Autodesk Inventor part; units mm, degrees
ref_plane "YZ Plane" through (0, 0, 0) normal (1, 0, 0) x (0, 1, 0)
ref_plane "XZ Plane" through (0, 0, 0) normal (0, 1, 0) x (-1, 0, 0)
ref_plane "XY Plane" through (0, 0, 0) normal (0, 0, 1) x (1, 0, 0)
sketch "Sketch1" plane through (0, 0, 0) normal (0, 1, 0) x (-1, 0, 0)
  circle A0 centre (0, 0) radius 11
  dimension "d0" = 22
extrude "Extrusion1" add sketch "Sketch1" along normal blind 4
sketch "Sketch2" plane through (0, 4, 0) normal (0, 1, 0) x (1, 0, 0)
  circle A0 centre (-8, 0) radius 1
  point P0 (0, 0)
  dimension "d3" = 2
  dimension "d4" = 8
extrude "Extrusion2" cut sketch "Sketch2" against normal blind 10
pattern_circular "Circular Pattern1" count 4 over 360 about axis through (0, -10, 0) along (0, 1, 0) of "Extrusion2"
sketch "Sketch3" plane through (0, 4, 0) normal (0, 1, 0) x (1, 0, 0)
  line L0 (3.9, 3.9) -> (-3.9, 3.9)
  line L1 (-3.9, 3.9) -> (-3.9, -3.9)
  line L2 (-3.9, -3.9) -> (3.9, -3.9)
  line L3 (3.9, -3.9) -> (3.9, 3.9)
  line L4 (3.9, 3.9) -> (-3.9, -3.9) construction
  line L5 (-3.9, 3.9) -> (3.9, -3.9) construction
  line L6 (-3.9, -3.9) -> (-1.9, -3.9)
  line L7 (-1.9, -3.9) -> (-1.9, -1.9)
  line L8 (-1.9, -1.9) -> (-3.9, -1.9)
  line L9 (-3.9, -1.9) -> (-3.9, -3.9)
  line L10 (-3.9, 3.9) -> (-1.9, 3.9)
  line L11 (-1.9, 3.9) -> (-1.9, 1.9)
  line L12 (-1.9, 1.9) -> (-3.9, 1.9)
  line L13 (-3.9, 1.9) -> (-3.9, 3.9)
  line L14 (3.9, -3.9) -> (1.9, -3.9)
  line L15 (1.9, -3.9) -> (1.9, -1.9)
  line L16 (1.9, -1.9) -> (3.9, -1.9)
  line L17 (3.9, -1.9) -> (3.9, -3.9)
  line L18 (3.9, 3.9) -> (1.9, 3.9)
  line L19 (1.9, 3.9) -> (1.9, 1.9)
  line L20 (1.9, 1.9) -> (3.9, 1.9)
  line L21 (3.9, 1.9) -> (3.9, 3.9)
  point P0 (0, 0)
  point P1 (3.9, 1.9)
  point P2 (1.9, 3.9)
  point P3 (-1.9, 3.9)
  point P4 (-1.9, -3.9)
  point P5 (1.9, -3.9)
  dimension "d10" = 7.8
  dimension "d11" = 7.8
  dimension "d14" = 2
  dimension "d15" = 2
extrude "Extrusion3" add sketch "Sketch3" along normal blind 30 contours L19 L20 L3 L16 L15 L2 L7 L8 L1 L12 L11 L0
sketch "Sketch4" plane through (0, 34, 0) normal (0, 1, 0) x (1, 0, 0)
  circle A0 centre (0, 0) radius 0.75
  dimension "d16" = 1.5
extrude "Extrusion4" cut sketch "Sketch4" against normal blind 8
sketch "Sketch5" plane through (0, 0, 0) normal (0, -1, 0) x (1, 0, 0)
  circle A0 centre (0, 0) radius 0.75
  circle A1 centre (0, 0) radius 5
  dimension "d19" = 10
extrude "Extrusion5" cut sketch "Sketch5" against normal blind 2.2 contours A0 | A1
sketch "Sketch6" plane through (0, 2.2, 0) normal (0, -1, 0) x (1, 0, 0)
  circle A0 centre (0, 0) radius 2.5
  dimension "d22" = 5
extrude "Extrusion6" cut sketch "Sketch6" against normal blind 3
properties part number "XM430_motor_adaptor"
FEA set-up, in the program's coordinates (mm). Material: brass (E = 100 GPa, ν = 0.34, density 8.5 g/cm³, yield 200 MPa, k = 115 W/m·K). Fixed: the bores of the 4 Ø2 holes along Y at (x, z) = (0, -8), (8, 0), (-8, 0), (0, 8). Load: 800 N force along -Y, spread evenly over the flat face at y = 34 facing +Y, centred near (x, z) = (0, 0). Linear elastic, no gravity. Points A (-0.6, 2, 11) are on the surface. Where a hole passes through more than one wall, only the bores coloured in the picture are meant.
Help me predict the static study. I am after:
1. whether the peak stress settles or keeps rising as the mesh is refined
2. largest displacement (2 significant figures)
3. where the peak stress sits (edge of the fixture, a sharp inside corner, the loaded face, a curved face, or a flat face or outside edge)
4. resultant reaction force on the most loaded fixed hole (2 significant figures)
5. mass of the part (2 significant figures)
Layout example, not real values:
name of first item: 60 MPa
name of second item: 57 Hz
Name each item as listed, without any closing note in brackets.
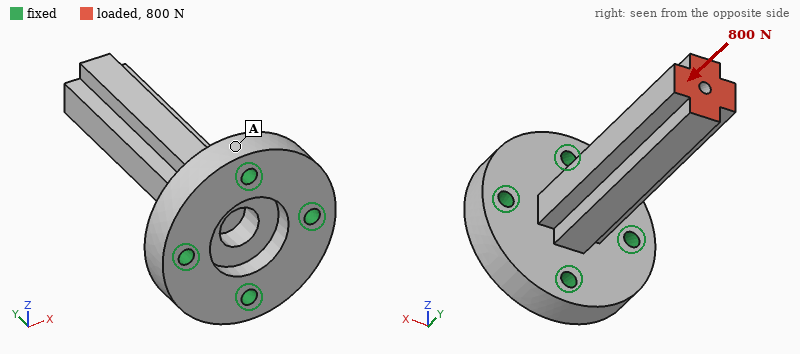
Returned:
whether the peak stress settles or keeps rising as the mesh is refined: keeps rising
largest displacement: 8.4 µm
where the peak stress sits: edge of the fixture
resultant reaction force on the most loaded fixed hole: 230 N
mass of the part: 22 g
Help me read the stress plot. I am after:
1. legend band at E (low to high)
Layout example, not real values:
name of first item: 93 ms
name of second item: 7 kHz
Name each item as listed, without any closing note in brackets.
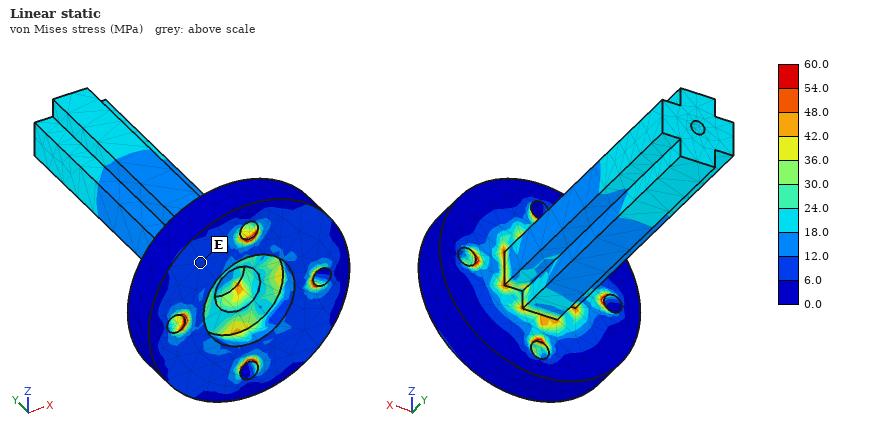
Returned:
legend band at E: 6.0 to 12.0 MPa
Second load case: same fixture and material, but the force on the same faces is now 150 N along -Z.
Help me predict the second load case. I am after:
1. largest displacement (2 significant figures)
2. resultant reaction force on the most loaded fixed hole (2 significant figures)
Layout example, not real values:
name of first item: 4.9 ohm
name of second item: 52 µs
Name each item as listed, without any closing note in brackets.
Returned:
largest displacement: 0.13 mm
resultant reaction force on the most loaded fixed hole: 390 N
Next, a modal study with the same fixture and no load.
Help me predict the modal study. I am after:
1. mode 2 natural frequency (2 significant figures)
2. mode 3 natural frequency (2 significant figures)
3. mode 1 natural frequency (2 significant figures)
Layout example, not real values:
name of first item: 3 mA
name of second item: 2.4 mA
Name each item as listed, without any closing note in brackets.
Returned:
mode 2 natural frequency: 3100 Hz
mode 3 natural frequency: 14 kHz
mode 1 natural frequency: 3100 Hz
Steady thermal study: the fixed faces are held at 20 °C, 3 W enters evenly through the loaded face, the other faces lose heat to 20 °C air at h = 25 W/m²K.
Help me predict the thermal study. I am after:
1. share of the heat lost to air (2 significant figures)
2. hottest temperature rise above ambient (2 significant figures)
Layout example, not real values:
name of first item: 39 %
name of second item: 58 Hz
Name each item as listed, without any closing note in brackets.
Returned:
share of the heat lost to air: 9.4 %
hottest temperature rise above ambient: 19 K
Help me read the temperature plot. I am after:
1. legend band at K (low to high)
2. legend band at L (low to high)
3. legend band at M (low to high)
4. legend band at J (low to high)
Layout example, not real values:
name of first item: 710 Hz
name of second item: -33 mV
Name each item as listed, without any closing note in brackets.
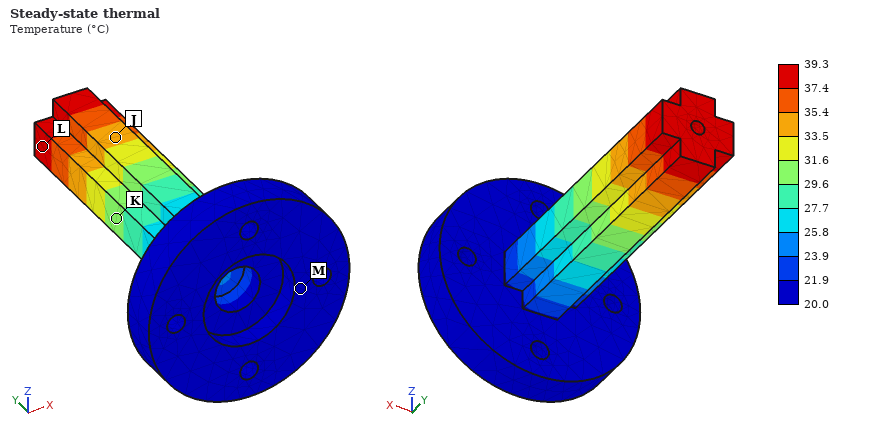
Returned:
legend band at K: 29.6 to 31.6 °C
legend band at L: 37.4 to 39.3 °C
legend band at M: 20.0 to 21.9 °C
legend band at J: 33.5 to 35.4 °C
